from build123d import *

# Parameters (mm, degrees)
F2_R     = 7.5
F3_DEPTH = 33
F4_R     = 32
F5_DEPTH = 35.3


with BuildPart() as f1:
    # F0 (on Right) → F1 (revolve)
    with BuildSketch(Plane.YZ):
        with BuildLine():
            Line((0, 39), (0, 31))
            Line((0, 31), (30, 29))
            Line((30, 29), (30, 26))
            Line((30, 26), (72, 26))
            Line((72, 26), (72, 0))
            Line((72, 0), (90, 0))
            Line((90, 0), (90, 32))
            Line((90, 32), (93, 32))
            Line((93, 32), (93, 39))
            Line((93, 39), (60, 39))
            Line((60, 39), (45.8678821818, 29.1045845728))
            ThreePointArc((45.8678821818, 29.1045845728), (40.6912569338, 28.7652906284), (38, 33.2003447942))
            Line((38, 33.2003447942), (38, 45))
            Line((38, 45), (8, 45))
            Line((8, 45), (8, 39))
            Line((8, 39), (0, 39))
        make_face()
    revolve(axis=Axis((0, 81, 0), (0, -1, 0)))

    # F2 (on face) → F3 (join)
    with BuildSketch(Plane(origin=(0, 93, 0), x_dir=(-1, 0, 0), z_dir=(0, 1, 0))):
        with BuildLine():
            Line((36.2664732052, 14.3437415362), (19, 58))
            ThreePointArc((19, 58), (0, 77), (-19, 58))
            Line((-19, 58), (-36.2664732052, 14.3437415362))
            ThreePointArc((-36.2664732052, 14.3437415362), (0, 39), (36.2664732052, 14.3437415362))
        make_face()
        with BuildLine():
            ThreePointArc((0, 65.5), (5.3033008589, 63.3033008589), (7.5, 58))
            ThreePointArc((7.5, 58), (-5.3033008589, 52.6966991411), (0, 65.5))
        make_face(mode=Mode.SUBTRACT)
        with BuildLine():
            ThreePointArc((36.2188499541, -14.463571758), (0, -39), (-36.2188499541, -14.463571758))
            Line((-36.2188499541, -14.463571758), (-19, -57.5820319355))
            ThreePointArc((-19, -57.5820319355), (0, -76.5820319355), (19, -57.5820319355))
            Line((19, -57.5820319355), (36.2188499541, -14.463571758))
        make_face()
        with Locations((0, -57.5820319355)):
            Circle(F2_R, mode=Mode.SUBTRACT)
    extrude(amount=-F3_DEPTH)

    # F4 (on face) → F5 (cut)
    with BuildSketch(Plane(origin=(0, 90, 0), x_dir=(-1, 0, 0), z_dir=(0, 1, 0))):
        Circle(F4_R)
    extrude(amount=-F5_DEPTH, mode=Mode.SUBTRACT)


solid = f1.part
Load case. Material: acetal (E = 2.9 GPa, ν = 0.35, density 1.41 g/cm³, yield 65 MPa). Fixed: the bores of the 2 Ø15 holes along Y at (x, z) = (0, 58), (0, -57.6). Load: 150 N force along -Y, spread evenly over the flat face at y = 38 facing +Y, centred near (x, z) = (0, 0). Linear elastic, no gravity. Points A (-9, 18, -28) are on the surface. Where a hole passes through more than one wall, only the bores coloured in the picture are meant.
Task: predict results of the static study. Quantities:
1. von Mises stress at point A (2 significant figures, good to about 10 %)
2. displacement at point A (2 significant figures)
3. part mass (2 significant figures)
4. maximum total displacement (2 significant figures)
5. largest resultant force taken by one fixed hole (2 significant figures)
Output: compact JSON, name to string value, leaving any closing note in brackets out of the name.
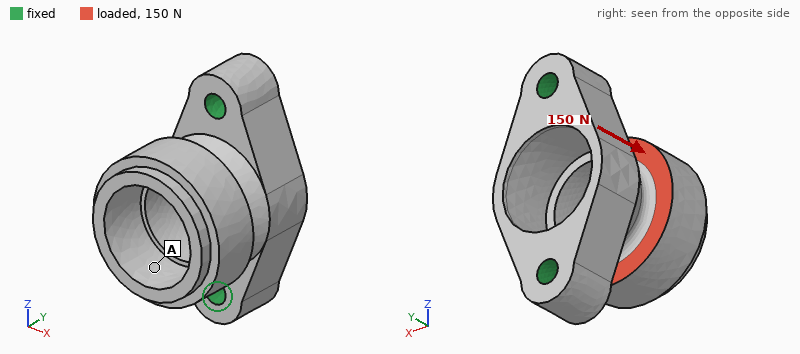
{"von Mises stress at point A": "0.12 MPa", "displacement at point A": "9.2 µm", "part mass": "420 g", "maximum total displacement": "12 µm", "largest resultant force taken by one fixed hole": "79 N"}
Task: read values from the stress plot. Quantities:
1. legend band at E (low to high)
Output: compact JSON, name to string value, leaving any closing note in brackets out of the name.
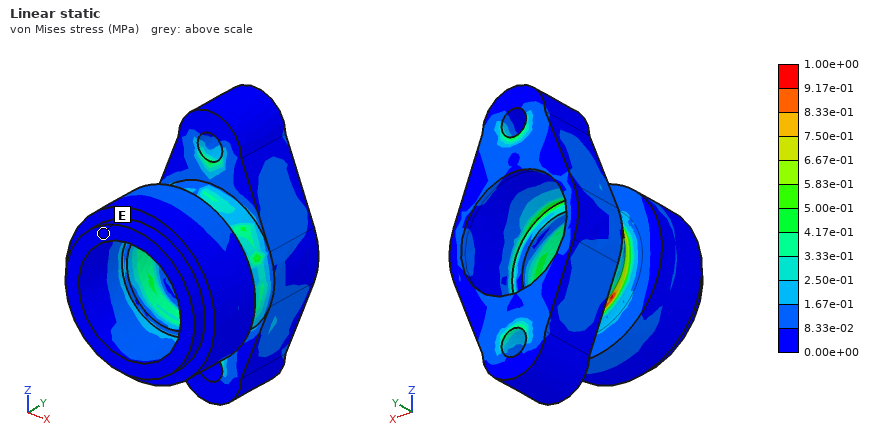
{"legend band at E": "0.00e+00 to 8.33e-02 MPa"}
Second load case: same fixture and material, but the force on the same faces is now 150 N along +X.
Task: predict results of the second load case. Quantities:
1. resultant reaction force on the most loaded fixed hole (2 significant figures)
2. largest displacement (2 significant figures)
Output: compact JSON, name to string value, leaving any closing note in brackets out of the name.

{"resultant reaction force on the most loaded fixed hole": "75 N", "largest displacement": "34 µm"}
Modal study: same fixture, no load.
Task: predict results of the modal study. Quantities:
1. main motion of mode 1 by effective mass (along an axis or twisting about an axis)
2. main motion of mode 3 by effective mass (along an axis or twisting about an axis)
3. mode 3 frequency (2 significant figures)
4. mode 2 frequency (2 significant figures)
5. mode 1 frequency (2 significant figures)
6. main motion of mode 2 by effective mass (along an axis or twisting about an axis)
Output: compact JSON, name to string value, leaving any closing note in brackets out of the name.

{"main motion of mode 1 by effective mass": "along X", "main motion of mode 3 by effective mass": "twisting about Y", "mode 3 frequency": "1300 Hz", "mode 2 frequency": "910 Hz", "mode 1 frequency": "620 Hz", "main motion of mode 2 by effective mass": "along Z"}
